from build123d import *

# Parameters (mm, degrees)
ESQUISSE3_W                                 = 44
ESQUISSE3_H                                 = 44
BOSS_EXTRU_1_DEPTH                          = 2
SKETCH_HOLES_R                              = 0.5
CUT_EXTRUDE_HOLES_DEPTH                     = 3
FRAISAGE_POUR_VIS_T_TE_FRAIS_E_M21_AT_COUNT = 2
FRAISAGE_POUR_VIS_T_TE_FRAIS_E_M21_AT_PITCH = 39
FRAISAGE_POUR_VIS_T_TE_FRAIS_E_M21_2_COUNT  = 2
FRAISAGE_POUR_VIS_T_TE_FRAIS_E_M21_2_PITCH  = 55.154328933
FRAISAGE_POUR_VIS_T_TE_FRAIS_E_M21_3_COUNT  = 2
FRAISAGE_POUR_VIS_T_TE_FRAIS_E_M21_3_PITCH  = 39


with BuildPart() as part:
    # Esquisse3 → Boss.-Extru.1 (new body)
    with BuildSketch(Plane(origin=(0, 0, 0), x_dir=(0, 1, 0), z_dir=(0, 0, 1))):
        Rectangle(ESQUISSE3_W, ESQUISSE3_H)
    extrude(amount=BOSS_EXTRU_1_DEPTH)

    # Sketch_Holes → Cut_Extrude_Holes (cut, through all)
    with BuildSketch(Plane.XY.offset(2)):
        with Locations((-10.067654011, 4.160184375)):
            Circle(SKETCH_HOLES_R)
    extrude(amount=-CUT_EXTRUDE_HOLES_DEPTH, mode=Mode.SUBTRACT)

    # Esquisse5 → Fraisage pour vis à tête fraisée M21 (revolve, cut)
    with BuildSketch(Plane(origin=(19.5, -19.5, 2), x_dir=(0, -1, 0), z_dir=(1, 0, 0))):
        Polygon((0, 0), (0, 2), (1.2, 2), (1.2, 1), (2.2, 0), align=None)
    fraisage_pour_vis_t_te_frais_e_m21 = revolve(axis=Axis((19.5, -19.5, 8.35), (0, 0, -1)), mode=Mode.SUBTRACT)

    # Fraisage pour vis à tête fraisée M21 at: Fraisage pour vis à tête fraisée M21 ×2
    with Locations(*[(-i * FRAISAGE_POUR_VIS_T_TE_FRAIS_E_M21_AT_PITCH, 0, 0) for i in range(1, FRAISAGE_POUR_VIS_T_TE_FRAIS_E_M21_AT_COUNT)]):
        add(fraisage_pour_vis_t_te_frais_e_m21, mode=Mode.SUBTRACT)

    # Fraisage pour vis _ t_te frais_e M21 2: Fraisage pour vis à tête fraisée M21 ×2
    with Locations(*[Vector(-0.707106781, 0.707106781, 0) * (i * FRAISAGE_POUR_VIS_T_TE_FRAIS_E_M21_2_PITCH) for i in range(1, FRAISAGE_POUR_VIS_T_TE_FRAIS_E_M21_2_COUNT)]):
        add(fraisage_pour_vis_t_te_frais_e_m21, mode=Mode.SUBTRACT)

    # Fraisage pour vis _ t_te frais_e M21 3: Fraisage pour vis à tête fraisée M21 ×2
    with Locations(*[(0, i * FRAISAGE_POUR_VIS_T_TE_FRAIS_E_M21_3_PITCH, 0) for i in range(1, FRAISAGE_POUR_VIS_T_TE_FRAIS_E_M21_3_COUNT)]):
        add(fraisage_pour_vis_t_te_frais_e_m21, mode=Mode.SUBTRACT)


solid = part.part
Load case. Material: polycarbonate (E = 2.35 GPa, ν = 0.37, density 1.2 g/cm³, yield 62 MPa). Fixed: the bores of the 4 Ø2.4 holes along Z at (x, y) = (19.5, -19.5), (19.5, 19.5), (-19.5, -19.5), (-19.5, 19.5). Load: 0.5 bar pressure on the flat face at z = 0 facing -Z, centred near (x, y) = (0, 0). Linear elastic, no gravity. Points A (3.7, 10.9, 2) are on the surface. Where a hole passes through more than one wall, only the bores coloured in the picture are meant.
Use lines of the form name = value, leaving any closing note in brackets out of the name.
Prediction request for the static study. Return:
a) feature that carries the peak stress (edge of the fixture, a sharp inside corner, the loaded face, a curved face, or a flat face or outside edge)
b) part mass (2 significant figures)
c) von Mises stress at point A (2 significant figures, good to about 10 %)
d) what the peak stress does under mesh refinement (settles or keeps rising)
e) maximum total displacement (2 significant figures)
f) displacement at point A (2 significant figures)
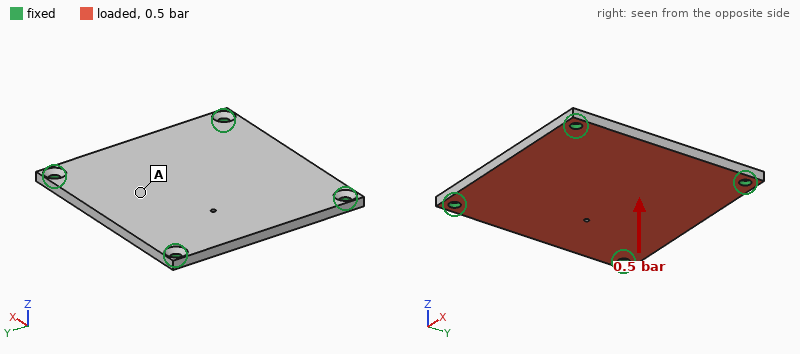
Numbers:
feature that carries the peak stress = edge of the fixture
part mass = 4.6 g
von Mises stress at point A = 6.9 MPa
what the peak stress does under mesh refinement = keeps rising
maximum total displacement = 0.64 mm
displacement at point A = 0.52 mm
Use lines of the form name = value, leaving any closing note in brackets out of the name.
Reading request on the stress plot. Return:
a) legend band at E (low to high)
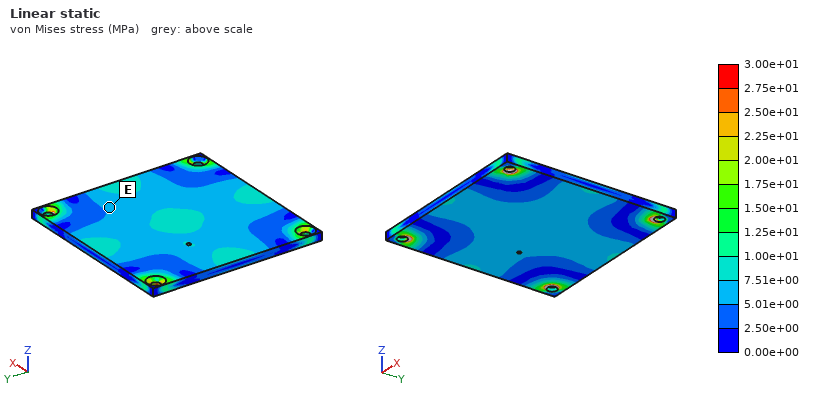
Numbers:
legend band at E = 5.01e+00 to 7.51e+00 MPa
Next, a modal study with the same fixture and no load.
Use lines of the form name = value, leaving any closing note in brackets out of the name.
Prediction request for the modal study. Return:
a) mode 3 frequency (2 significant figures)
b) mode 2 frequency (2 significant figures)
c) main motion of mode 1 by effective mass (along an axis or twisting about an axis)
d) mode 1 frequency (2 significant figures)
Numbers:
mode 3 frequency = 1900 Hz
mode 2 frequency = 1900 Hz
main motion of mode 1 by effective mass = along Z
mode 1 frequency = 1100 Hz
